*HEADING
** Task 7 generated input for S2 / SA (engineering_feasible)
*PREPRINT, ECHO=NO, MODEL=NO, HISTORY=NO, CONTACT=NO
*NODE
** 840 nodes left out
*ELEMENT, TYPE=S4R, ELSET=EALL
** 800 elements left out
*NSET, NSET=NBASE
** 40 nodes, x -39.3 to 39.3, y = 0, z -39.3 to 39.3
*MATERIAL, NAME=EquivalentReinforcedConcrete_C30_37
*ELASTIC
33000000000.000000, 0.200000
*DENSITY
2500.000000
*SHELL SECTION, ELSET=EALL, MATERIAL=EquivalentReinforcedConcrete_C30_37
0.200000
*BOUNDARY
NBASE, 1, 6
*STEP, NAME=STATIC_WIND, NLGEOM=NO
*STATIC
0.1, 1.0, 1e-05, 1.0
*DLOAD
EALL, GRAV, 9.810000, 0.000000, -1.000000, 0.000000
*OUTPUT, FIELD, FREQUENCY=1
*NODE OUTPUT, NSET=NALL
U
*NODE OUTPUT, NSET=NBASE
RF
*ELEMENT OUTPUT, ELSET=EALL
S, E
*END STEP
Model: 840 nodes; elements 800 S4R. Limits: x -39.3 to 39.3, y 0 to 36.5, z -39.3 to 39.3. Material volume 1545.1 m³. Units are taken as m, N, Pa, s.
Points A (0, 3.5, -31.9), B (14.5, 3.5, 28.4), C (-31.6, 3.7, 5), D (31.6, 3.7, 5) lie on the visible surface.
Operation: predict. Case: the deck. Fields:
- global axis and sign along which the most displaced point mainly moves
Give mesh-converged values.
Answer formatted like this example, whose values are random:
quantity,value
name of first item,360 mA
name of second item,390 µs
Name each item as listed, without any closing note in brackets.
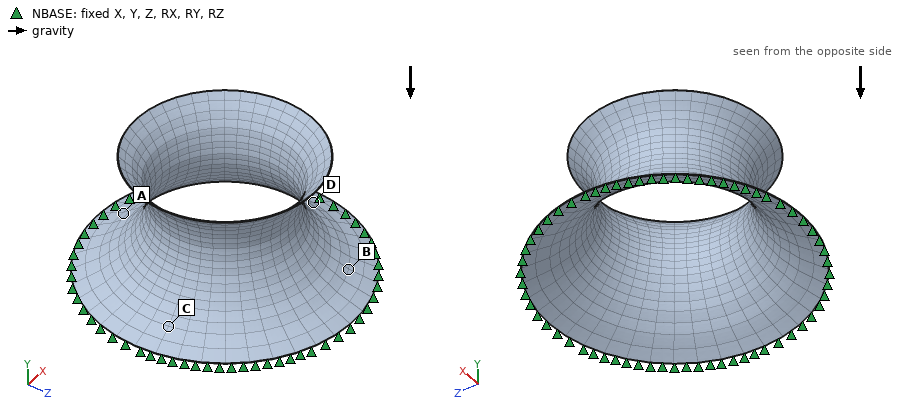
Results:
quantity,value
global axis and sign along which the most displaced point mainly moves,-Y
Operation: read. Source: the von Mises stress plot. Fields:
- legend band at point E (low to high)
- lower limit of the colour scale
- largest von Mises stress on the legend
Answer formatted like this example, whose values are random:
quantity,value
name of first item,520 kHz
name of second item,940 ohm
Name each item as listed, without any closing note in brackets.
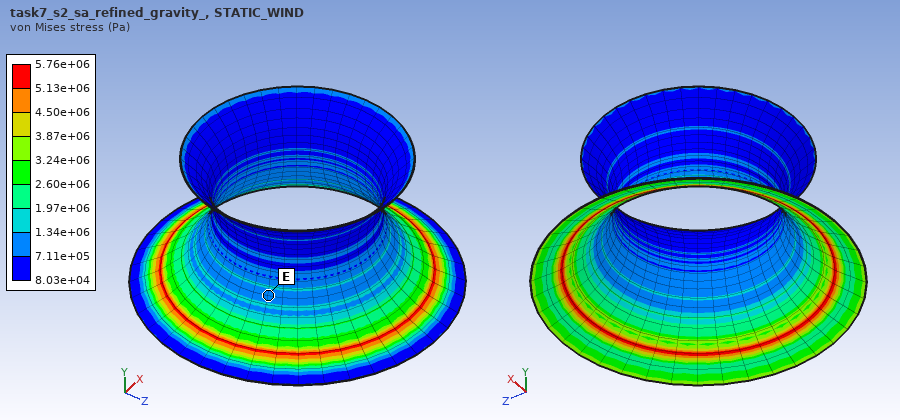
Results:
quantity,value
legend band at point E,7.11e+05 to 1.34e+06 Pa
lower limit of the colour scale,8.03e+04 Pa
largest von Mises stress on the legend,5.76e+06 Pa
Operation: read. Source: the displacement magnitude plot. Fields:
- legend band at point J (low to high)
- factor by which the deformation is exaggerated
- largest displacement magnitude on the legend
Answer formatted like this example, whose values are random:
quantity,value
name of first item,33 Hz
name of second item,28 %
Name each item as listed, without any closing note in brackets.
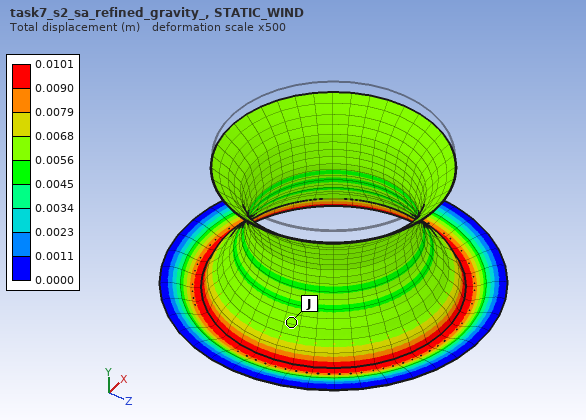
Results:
quantity,value
legend band at point J,0.0056 to 0.0068 m
factor by which the deformation is exaggerated,500
largest displacement magnitude on the legend,0.0101 m
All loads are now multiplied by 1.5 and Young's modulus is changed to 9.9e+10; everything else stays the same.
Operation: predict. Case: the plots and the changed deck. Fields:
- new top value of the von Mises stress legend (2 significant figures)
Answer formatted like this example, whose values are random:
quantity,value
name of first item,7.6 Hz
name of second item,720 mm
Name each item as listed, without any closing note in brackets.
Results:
quantity,value
new top value of the von Mises stress legend,8.6e+06 Pa
